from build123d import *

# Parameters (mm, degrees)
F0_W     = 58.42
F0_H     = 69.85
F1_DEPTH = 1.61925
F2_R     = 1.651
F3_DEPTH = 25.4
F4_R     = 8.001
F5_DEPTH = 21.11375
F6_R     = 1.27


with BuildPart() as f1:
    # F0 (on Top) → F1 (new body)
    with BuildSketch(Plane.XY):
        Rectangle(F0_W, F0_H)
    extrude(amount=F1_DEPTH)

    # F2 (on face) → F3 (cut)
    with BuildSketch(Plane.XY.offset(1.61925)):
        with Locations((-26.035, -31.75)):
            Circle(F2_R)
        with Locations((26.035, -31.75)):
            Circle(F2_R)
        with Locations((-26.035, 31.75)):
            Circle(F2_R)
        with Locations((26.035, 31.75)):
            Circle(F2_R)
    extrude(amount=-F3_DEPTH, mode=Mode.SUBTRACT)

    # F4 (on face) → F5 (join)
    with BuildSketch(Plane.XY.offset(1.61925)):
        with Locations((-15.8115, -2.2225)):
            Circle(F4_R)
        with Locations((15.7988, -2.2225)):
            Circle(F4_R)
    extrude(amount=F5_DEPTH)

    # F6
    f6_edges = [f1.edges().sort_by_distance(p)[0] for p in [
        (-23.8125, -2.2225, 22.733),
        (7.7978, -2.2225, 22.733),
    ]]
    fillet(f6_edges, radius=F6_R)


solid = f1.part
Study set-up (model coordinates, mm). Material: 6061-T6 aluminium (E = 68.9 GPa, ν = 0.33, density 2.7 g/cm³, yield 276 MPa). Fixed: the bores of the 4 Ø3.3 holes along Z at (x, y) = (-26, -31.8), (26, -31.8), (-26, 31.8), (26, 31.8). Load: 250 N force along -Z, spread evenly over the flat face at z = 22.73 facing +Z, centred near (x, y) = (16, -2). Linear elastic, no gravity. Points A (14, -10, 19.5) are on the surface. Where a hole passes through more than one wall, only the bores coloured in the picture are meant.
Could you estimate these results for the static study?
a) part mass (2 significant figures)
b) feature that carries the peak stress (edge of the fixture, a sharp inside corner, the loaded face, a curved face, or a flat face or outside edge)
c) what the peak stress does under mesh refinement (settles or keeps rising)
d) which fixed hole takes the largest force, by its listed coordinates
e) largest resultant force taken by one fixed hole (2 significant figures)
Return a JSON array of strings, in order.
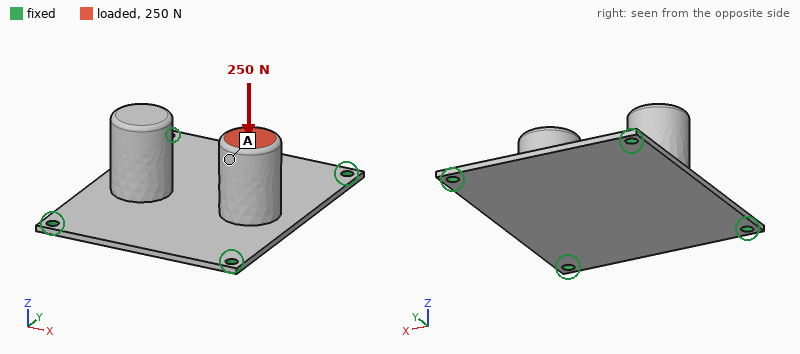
["41 g", "edge of the fixture", "keeps rising", "(26, -31.8)", "120 N"]
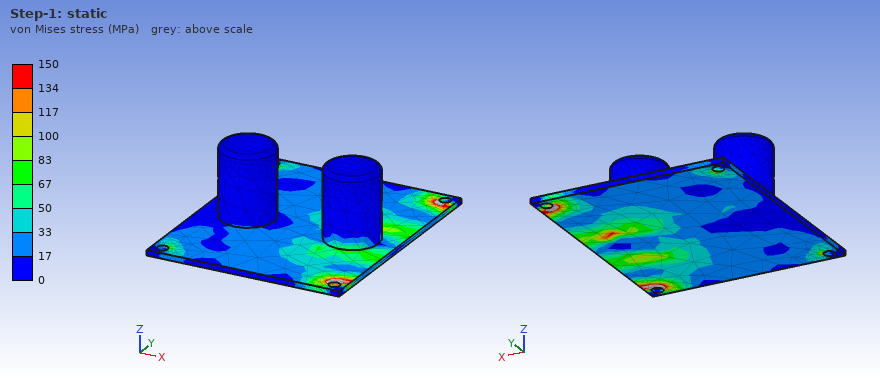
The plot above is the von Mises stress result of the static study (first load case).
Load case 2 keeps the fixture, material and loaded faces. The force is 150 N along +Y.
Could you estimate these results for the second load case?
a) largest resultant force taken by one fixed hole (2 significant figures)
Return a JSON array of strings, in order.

["76 N"]
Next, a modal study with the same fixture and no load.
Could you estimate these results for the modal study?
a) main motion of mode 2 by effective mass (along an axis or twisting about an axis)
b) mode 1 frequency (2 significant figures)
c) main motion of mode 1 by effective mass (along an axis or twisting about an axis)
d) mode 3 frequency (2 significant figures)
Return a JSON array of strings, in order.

["along X", "960 Hz", "along Z", "1400 Hz"]
